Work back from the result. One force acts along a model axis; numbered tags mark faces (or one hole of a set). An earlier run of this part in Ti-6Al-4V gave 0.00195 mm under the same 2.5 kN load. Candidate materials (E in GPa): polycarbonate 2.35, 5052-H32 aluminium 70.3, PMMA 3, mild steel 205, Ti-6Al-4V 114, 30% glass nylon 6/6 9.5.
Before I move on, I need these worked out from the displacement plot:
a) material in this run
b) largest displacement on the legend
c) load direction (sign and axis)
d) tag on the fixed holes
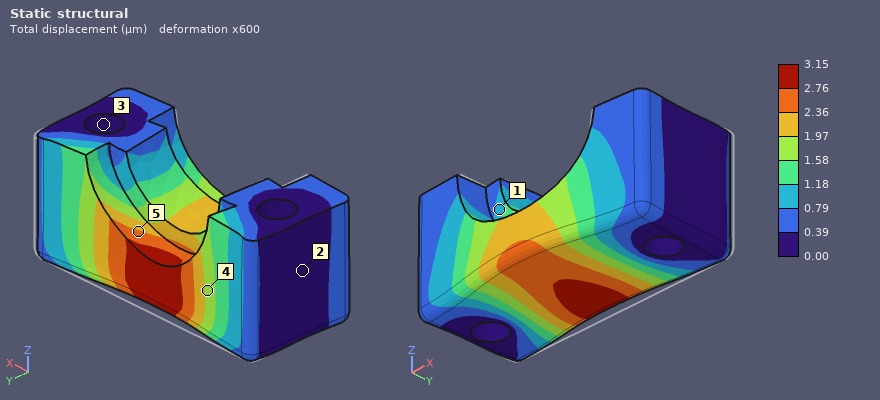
5052-H32 aluminium
3.15 µm
-Y
3
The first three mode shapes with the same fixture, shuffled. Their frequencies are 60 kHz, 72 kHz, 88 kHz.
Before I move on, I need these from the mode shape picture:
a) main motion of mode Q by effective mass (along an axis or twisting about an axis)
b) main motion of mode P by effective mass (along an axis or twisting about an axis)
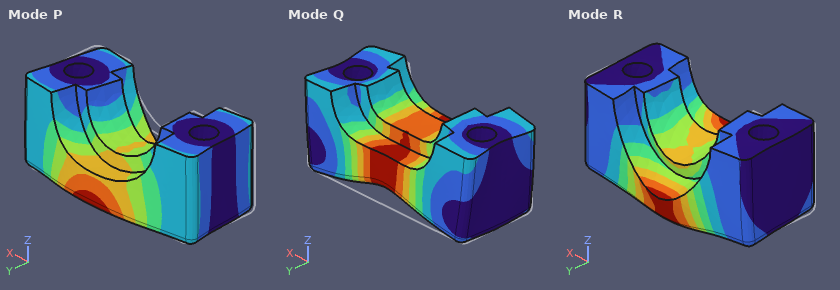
along Z
along Y
